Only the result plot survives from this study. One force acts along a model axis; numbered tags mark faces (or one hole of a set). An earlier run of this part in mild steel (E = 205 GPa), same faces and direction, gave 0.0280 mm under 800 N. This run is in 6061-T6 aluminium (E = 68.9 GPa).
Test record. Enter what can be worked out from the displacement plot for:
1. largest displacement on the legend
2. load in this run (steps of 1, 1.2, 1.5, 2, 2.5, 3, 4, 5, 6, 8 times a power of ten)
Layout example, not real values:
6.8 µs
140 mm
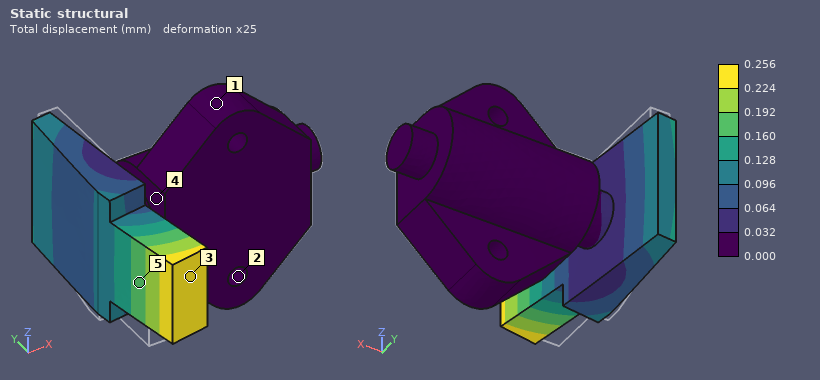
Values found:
0.256 mm
2.5 kN
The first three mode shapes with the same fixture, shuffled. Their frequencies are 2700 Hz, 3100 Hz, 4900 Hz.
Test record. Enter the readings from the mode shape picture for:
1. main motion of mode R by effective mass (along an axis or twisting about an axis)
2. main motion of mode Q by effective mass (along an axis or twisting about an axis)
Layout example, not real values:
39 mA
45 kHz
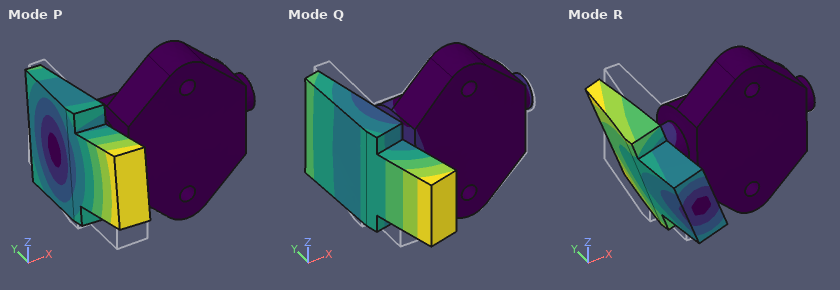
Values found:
along Z
along Y
